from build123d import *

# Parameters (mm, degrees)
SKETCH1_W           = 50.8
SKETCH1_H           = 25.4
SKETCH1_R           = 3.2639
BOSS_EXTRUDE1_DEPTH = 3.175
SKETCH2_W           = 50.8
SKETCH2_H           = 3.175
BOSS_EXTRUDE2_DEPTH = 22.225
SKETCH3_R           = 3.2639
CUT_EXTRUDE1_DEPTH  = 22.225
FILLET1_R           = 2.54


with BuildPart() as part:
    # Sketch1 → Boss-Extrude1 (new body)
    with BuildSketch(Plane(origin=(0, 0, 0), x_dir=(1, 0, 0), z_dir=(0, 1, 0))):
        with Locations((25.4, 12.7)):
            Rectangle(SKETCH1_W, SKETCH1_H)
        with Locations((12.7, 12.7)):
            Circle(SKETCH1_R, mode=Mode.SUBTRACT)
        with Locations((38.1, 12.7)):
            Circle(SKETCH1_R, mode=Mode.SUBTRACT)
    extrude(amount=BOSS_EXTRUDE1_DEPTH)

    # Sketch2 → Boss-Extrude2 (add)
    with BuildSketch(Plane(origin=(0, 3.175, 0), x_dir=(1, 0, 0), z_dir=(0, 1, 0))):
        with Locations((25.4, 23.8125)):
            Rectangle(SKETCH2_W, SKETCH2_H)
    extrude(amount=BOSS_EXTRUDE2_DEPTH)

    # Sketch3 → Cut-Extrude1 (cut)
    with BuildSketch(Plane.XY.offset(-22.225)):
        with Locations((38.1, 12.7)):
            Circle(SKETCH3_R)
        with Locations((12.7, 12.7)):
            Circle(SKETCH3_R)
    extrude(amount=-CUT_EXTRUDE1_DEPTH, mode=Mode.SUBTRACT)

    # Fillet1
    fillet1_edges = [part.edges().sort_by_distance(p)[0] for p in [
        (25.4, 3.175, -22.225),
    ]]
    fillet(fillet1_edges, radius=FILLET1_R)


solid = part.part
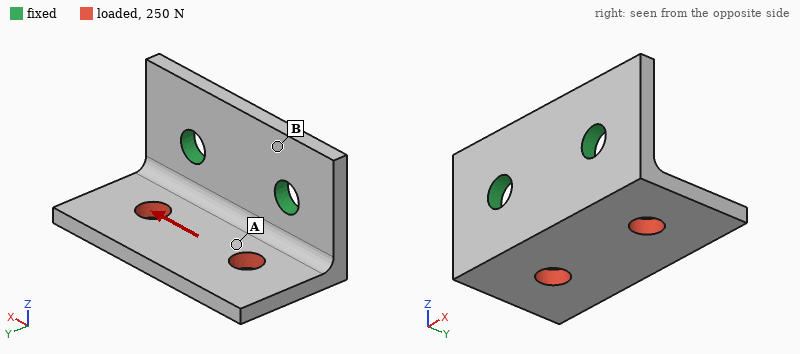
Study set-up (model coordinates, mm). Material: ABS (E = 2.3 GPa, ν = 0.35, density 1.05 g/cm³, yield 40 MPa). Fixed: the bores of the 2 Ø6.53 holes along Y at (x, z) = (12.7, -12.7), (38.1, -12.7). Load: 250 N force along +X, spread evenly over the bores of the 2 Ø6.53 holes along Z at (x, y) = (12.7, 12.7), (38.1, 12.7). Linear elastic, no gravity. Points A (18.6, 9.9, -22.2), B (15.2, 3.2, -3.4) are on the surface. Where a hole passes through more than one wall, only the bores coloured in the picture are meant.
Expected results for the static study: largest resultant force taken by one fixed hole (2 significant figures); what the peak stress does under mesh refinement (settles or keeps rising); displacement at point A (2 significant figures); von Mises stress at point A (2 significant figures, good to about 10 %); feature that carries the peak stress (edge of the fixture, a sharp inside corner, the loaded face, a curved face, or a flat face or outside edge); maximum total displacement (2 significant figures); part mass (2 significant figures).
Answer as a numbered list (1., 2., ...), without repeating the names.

1. 170 N
2. keeps rising
3. 0.14 mm
4. 6.5 MPa
5. edge of the fixture
6. 0.45 mm
7. 7.7 g
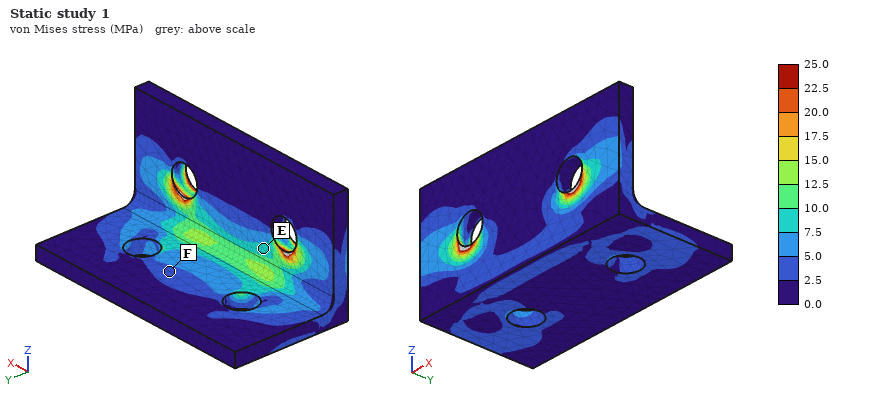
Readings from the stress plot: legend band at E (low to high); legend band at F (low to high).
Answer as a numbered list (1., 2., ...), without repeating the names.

1. 7.5 to 10.0 MPa
2. 2.5 to 5.0 MPa
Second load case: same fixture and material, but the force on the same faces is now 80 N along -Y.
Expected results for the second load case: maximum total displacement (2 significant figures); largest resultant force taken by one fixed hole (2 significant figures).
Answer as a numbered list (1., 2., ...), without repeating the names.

1. 0.29 mm
2. 40 N
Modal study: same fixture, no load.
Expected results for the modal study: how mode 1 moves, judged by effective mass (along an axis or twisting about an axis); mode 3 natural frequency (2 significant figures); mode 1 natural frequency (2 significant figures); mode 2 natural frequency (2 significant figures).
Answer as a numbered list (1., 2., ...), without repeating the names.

1. along Z
2. 2600 Hz
3. 910 Hz
4. 1500 Hz
